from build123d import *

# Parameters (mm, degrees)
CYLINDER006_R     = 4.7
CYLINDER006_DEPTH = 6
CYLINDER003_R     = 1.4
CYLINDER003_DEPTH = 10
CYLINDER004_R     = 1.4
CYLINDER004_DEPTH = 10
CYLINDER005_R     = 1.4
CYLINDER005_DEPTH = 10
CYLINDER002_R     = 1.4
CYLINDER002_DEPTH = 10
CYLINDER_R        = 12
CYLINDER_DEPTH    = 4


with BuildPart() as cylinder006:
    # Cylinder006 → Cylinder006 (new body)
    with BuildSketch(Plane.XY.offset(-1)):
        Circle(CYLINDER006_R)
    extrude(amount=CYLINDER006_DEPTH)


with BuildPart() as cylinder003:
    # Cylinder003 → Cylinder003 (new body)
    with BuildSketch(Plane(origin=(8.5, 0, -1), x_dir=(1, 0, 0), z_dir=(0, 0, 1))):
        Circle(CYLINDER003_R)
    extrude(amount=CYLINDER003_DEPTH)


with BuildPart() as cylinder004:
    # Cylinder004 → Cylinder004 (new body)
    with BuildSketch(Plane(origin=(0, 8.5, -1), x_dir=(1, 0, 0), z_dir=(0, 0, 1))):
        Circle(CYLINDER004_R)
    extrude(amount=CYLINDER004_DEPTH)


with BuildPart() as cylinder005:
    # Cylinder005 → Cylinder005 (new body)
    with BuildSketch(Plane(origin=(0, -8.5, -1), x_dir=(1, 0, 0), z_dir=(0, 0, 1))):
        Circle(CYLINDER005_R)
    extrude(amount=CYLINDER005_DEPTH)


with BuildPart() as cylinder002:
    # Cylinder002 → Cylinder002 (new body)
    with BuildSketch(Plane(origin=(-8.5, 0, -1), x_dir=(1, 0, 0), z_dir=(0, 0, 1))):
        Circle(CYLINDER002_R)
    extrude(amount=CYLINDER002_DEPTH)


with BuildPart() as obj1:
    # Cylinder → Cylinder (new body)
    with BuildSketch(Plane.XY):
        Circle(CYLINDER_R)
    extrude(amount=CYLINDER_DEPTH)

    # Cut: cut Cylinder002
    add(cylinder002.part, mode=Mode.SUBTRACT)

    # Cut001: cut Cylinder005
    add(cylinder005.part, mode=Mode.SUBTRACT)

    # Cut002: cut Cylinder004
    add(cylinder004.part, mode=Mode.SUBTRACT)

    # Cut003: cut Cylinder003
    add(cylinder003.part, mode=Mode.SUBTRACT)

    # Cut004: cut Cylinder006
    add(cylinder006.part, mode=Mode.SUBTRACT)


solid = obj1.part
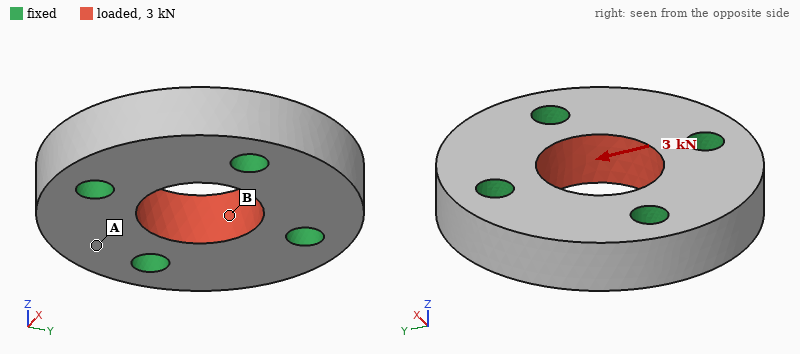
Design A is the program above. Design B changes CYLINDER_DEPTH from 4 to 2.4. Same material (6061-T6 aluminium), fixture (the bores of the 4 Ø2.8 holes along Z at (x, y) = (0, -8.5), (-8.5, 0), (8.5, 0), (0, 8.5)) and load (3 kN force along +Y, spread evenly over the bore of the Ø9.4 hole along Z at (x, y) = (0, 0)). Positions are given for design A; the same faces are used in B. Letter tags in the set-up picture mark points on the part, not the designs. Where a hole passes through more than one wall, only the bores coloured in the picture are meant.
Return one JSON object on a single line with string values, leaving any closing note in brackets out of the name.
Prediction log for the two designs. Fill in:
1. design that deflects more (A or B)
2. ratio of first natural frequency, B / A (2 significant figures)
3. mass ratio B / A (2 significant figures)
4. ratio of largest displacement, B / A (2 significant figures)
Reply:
{"design that deflects more": "B", "ratio of first natural frequency, B / A": "0.75", "mass ratio B / A": "0.60", "ratio of largest displacement, B / A": "1.7"}
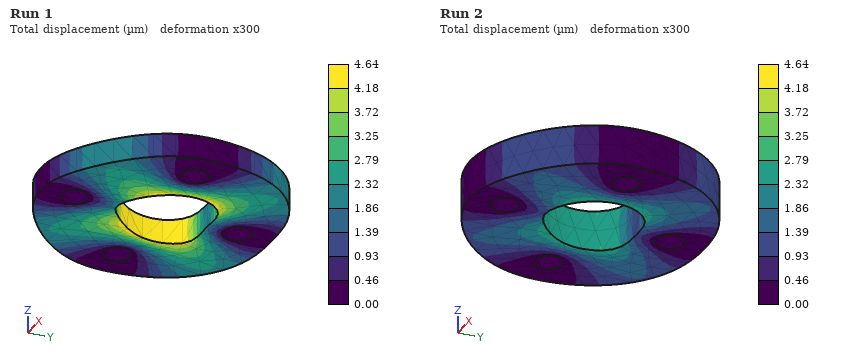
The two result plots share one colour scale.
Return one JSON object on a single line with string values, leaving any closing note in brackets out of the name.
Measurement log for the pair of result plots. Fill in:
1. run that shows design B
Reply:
{"run that shows design B": "Run 1"}
